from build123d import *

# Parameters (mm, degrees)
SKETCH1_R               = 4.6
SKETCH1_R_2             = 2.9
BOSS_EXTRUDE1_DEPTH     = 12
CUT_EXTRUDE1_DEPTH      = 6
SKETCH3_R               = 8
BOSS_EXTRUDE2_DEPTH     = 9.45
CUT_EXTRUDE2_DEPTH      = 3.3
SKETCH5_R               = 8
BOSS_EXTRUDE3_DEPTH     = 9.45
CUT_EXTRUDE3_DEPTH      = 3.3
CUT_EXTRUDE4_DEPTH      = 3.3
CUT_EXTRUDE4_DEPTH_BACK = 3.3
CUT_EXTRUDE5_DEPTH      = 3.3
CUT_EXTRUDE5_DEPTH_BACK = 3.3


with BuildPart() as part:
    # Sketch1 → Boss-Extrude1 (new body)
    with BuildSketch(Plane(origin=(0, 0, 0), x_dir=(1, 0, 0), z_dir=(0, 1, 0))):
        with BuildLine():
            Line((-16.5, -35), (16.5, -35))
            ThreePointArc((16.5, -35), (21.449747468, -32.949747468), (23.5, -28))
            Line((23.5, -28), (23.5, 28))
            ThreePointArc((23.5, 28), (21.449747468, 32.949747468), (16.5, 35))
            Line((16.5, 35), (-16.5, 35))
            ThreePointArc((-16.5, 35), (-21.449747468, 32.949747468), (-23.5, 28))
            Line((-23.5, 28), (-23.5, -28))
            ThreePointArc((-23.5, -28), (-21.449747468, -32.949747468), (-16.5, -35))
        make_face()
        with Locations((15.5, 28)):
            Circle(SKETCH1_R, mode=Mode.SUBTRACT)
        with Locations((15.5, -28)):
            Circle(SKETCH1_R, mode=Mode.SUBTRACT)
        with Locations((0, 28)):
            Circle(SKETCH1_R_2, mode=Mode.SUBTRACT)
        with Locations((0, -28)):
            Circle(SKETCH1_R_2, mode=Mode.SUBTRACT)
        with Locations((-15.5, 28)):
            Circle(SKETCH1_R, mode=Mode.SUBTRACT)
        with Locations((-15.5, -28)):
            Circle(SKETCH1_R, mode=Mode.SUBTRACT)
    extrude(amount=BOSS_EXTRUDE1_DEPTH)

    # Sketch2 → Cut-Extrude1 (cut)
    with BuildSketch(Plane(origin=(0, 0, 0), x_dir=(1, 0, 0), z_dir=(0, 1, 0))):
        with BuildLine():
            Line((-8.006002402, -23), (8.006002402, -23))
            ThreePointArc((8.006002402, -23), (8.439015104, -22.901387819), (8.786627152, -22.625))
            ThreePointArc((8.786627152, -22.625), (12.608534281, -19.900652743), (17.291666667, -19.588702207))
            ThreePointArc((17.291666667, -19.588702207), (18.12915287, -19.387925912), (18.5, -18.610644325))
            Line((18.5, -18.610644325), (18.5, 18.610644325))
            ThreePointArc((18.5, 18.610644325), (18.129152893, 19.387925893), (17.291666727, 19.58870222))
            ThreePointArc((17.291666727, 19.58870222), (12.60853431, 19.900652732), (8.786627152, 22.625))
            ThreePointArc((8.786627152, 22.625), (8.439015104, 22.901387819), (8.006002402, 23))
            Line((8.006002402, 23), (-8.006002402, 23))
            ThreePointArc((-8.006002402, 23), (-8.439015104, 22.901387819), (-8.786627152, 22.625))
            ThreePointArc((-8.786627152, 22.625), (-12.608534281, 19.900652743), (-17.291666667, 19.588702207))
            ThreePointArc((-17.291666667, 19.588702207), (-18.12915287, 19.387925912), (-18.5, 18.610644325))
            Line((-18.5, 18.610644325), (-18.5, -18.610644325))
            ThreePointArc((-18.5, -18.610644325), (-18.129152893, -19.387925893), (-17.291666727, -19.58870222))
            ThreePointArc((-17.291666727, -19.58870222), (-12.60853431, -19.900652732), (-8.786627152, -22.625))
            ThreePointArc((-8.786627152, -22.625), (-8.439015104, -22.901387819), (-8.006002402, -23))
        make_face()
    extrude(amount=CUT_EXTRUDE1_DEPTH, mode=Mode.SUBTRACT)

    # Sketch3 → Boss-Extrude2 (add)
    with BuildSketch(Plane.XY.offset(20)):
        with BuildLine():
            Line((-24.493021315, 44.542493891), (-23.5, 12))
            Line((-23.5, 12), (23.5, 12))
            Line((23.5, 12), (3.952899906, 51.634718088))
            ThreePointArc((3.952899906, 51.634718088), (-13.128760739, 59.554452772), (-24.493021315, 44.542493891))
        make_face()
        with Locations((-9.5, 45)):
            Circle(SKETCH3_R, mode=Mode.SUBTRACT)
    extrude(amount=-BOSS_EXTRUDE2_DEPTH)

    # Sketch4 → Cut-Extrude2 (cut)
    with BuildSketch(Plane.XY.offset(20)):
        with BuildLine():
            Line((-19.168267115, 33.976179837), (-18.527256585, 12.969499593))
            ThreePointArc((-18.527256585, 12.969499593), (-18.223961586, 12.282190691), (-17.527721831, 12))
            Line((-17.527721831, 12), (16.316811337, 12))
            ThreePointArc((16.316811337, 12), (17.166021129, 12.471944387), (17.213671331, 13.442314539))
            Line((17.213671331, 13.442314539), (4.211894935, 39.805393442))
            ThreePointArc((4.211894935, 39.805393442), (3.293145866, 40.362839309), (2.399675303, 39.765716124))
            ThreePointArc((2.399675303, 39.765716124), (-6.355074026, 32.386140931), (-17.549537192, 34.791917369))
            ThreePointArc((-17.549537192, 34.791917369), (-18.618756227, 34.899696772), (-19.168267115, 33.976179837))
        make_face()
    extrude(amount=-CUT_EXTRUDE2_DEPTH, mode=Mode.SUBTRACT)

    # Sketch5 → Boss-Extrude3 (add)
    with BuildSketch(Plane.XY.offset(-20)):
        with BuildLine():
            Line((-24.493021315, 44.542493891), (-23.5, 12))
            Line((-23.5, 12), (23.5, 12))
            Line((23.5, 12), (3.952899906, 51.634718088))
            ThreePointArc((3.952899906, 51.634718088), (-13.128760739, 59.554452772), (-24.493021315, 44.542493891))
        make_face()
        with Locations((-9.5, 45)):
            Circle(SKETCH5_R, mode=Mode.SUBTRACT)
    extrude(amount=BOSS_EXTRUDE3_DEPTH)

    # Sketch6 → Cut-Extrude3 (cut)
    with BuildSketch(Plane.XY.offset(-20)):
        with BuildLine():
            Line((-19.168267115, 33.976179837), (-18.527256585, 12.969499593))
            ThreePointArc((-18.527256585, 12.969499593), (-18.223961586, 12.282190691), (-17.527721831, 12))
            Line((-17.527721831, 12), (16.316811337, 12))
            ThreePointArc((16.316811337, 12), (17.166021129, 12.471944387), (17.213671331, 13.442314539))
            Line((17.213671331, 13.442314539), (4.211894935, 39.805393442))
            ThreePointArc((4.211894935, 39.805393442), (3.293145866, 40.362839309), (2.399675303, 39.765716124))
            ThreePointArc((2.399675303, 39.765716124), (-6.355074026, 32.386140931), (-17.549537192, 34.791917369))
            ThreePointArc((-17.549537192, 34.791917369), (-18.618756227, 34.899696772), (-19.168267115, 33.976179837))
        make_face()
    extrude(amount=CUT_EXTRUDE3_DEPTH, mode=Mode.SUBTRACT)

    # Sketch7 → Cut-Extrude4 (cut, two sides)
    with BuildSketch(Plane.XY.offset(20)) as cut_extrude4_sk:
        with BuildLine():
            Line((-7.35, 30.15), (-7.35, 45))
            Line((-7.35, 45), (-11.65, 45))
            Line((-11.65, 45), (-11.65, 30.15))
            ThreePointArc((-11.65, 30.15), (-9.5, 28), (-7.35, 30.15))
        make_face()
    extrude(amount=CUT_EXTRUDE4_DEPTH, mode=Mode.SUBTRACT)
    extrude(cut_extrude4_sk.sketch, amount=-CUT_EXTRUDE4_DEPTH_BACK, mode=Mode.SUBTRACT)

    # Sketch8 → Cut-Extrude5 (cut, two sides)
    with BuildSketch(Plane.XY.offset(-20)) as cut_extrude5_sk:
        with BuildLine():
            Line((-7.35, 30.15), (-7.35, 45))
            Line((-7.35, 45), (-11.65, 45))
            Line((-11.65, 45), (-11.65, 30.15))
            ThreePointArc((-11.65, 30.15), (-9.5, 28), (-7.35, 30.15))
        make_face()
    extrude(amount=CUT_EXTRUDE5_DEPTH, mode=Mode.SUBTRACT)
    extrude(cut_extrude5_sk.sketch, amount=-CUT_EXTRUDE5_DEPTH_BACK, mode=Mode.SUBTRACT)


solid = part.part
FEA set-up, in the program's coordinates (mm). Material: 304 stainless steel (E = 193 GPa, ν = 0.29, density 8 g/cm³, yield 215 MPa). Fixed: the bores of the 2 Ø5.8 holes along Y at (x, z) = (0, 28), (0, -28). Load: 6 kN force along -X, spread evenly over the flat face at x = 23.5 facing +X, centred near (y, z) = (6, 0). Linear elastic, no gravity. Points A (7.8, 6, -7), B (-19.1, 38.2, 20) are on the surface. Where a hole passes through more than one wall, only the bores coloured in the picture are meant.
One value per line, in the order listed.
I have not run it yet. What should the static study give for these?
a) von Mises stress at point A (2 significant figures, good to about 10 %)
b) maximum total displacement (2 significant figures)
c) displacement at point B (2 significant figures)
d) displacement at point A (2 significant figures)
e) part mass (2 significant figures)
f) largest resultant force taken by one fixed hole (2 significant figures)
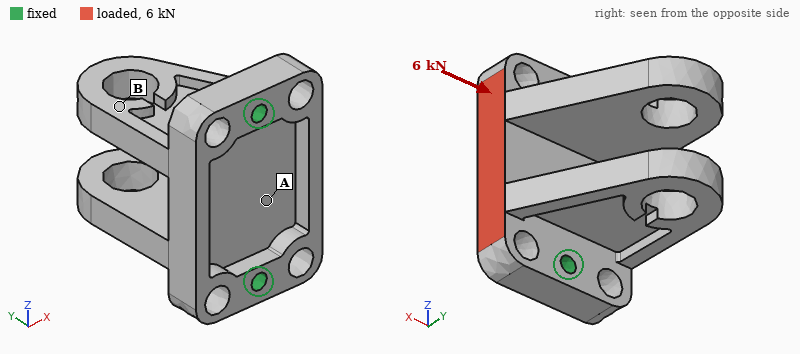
17 MPa
11 µm
2.7 µm
3.3 µm
390 g
3.1 kN
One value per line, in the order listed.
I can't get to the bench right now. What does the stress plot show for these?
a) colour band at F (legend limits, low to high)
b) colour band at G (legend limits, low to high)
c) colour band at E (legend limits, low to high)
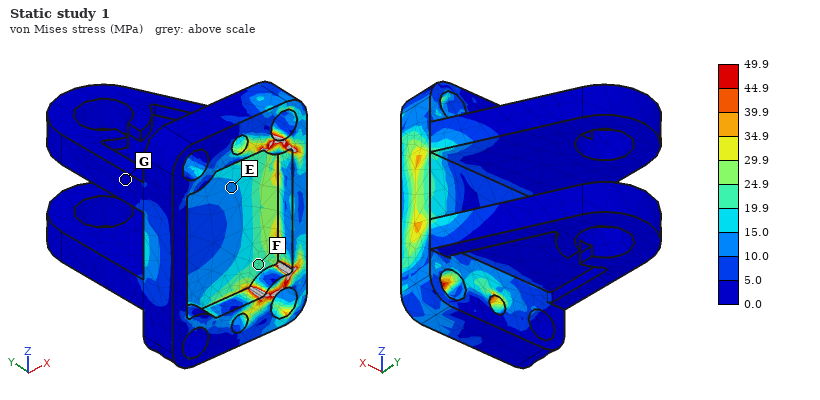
19.9 to 24.9 MPa
0.0 to 5.0 MPa
10.0 to 15.0 MPa
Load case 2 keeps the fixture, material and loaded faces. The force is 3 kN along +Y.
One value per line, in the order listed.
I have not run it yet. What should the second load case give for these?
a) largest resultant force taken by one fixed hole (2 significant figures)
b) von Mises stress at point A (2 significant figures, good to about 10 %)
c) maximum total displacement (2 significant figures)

1.6 kN
20 MPa
35 µm
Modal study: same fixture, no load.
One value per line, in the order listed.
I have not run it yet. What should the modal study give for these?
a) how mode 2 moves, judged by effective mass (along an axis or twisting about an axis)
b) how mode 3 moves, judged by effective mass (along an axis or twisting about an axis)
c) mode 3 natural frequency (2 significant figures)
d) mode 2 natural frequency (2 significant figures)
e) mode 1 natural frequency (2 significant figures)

along Z
along X
3400 Hz
2800 Hz
2400 Hz
